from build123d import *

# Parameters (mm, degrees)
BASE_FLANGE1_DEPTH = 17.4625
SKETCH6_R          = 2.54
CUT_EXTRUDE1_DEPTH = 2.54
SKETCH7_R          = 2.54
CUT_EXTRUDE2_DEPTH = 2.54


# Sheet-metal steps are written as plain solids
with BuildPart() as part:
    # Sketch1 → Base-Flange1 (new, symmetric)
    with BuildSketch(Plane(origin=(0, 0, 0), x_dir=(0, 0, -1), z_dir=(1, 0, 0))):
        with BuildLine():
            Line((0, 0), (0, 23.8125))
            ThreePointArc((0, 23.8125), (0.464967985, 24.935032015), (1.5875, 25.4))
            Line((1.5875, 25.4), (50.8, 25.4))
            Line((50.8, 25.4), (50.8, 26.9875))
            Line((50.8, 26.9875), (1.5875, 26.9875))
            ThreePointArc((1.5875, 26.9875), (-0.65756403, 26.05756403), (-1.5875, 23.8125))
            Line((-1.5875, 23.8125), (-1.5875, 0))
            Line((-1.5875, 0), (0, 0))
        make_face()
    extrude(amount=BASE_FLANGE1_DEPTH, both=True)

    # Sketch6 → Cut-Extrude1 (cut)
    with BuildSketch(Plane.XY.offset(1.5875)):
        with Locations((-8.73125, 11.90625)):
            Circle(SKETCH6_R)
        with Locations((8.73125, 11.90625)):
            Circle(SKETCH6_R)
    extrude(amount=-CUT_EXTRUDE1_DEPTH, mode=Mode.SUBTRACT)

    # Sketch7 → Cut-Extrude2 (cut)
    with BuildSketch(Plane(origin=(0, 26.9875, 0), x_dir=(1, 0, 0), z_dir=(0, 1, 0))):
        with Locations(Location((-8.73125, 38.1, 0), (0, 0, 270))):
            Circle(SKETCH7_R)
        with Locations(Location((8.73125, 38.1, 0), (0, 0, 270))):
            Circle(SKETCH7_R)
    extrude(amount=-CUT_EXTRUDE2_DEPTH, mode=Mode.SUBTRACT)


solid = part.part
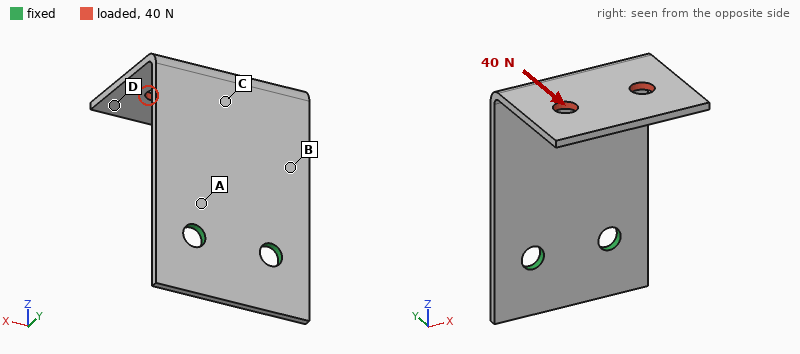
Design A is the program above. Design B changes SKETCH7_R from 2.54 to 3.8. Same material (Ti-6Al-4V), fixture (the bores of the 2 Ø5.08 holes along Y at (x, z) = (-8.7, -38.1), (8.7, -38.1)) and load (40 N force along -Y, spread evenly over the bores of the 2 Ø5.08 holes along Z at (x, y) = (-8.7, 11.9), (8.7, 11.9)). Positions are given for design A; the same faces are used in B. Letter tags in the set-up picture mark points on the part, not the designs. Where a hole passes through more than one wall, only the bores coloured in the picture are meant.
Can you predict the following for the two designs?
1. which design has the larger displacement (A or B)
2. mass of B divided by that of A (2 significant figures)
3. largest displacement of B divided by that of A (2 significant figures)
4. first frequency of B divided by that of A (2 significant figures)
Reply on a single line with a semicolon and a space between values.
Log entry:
A; 0.98; 0.90; 1.1
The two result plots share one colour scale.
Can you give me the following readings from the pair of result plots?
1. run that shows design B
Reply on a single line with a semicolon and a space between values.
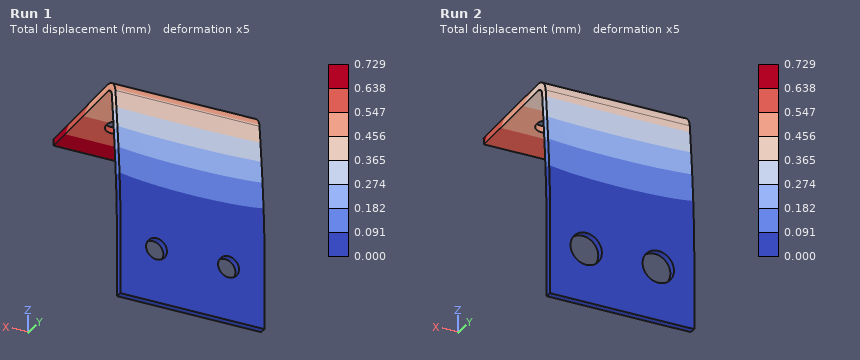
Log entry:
Run 2
